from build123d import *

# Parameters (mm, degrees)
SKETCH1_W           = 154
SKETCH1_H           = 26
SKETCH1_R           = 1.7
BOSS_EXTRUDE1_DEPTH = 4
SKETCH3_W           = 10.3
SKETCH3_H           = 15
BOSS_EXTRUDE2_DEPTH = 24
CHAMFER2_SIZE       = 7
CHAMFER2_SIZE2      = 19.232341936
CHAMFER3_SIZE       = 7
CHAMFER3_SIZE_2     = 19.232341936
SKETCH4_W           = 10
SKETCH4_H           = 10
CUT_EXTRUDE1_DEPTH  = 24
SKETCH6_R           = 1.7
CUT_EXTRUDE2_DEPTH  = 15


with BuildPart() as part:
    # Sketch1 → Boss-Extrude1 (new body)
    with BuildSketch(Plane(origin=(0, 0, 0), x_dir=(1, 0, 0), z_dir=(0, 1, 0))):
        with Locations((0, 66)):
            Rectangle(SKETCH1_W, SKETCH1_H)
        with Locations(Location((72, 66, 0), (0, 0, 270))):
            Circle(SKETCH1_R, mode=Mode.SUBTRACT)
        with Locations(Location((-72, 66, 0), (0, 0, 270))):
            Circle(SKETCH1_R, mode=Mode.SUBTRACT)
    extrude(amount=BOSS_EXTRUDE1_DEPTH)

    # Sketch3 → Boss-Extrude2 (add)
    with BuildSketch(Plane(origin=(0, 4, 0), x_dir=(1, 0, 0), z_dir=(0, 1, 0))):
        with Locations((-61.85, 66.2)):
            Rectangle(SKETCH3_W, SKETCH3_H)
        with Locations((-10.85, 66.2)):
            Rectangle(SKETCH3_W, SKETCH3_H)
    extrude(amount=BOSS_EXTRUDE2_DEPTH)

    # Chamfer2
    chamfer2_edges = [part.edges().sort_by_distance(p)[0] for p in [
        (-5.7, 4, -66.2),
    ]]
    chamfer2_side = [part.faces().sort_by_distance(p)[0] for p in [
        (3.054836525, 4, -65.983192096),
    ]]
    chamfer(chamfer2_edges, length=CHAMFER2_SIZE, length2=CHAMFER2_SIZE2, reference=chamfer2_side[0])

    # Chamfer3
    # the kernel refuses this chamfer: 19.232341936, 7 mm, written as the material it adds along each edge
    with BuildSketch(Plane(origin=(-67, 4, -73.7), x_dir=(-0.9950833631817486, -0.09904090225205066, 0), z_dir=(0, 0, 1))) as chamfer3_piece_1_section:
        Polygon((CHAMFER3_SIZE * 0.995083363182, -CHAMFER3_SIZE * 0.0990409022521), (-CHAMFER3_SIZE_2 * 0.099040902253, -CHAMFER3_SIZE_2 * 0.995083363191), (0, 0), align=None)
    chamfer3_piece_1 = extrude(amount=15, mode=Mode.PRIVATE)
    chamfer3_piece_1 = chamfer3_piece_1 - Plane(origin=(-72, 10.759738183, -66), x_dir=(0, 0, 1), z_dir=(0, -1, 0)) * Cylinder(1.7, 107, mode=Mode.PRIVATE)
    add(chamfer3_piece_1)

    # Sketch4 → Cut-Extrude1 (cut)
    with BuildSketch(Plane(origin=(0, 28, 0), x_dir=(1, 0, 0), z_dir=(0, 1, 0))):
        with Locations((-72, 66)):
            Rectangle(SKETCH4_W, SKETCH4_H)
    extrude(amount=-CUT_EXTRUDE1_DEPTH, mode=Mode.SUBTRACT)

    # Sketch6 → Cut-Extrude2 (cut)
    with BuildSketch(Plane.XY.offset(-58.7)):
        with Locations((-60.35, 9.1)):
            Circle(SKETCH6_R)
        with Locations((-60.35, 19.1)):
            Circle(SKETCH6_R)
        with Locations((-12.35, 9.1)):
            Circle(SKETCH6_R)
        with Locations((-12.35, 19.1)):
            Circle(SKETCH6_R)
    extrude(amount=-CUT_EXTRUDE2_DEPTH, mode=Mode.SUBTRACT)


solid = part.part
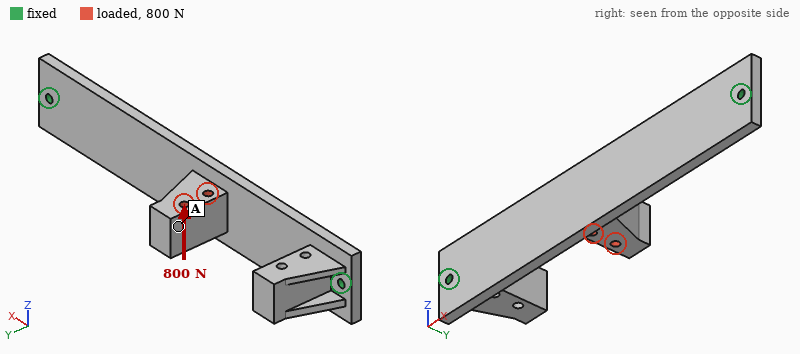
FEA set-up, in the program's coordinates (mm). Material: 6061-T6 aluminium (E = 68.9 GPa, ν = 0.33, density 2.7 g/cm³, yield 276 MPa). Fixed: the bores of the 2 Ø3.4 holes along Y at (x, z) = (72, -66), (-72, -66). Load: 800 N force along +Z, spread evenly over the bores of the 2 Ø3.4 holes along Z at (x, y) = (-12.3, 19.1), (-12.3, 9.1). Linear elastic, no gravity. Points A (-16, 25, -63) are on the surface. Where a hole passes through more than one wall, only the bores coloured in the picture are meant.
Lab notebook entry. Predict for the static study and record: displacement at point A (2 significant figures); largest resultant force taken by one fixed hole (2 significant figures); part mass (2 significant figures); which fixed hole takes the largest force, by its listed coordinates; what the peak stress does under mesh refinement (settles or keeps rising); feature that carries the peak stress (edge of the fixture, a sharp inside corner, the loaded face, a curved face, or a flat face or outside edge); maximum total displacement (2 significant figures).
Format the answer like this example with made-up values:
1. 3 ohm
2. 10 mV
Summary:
1. 0.56 mm
2. 480 N
3. 65 g
4. (-72, -66)
5. keeps rising
6. edge of the fixture
7. 0.64 mm
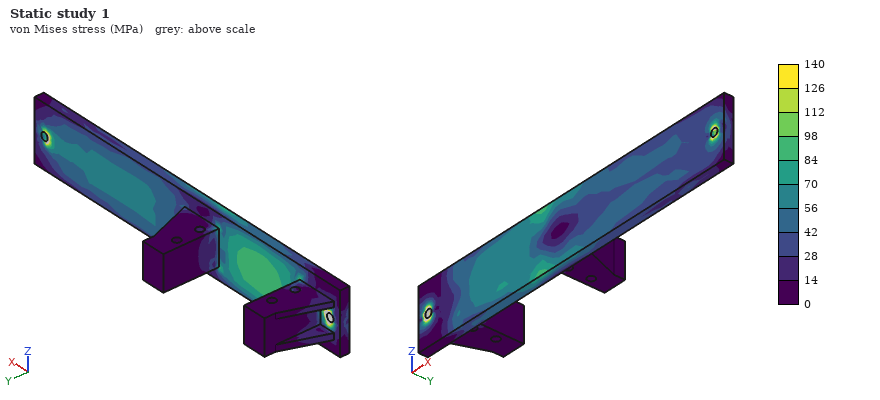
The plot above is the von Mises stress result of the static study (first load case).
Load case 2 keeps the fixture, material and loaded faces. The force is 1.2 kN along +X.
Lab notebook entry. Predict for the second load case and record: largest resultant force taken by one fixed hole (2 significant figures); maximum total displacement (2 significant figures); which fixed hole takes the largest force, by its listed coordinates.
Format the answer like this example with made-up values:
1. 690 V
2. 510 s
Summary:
1. 660 N
2. 0.29 mm
3. (-72, -66)
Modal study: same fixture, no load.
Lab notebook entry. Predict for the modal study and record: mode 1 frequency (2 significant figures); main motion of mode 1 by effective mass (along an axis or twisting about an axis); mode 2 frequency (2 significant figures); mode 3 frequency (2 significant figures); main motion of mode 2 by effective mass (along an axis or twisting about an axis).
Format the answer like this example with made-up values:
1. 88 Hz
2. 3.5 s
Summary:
1. 860 Hz
2. along Y
3. 1700 Hz
4. 2200 Hz
5. along Z
